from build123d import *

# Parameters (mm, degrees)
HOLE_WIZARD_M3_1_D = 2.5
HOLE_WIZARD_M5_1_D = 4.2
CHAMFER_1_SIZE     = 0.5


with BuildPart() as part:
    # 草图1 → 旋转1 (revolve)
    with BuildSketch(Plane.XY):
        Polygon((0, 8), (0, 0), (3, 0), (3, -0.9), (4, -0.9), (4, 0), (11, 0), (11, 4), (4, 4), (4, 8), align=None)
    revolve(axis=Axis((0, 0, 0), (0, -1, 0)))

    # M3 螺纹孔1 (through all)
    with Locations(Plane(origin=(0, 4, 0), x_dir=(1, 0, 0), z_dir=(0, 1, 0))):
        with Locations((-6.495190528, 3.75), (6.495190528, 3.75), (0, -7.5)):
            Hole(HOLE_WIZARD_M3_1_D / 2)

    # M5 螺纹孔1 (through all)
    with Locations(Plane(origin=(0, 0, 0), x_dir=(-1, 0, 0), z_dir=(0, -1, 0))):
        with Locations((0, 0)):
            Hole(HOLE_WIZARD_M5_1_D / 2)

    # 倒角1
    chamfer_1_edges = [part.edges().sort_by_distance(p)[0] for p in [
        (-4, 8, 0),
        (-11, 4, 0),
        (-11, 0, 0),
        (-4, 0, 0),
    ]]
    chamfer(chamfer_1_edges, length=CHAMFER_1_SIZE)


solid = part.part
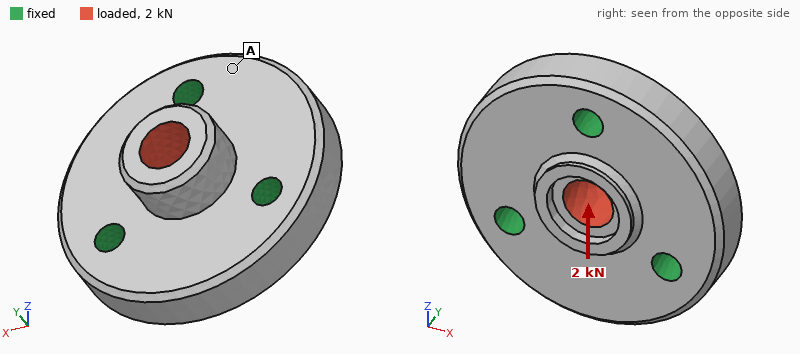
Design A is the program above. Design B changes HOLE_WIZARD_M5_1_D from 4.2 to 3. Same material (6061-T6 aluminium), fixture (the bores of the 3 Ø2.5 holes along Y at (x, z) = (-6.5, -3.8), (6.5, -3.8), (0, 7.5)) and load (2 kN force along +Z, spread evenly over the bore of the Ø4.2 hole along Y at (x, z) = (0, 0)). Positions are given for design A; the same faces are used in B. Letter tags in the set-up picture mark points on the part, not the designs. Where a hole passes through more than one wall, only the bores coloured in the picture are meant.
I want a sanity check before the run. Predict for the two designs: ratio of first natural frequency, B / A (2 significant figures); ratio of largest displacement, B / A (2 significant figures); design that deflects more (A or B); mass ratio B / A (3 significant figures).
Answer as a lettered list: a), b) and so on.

a) 1.0
b) 0.87
c) A
d) 1.03
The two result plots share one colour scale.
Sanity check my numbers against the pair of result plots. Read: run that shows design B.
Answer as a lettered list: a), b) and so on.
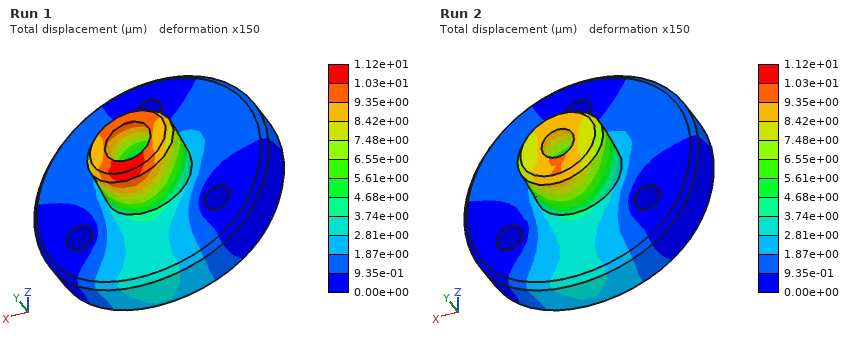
a) Run 2
